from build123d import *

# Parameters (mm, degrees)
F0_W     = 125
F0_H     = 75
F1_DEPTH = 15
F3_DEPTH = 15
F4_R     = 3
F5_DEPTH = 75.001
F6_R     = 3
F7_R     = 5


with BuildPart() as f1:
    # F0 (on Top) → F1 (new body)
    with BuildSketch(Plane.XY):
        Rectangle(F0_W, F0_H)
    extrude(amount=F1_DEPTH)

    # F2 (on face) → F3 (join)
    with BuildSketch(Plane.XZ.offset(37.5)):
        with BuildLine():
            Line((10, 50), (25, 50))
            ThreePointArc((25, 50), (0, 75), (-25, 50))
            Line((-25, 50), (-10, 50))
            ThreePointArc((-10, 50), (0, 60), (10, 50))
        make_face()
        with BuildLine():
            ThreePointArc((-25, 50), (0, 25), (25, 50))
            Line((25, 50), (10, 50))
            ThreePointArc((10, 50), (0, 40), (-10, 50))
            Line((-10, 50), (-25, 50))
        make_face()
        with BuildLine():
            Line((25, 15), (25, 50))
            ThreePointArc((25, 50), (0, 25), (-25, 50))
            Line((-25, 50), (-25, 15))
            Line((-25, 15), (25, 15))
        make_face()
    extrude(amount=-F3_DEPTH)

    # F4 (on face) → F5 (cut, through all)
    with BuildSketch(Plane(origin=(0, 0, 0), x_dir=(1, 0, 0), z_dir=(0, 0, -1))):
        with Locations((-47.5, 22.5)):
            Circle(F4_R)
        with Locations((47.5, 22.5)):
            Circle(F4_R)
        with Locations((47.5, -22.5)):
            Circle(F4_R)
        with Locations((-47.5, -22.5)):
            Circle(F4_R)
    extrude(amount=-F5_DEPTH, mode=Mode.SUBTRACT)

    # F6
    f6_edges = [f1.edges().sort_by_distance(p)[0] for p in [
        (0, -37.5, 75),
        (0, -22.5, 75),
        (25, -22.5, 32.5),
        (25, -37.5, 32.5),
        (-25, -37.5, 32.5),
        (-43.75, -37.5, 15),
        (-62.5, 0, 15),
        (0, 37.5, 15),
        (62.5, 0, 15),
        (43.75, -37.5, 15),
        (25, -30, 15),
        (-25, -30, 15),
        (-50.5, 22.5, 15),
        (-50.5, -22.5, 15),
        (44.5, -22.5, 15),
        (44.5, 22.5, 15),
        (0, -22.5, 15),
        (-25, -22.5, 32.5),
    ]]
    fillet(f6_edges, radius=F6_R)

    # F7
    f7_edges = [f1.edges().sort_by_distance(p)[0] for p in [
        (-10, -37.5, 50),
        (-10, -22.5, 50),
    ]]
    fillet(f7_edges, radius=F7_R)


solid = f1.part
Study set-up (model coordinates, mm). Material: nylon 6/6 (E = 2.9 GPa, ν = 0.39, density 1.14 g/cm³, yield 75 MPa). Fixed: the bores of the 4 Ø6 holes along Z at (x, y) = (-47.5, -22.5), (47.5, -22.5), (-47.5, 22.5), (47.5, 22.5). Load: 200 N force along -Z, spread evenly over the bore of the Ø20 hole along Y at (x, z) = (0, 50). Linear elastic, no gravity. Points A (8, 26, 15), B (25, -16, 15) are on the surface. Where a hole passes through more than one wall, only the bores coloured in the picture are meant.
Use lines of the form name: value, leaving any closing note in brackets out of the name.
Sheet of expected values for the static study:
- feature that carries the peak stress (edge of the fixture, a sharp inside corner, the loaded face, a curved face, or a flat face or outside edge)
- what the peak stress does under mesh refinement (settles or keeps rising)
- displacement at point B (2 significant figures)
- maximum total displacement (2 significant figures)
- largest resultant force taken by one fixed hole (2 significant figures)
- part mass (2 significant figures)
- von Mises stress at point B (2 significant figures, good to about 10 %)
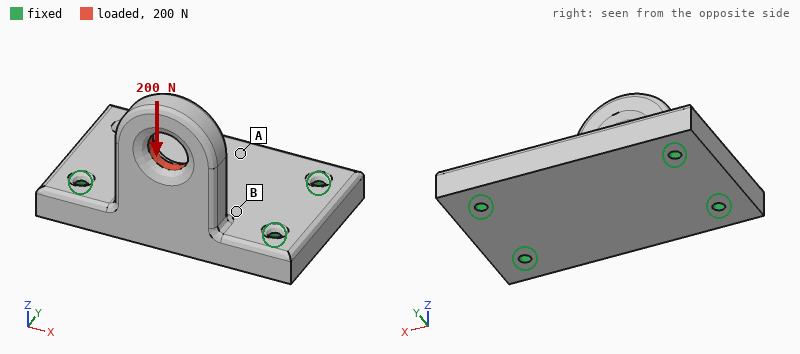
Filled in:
feature that carries the peak stress: edge of the fixture
what the peak stress does under mesh refinement: keeps rising
displacement at point B: 13 µm
maximum total displacement: 58 µm
largest resultant force taken by one fixed hole: 120 N
part mass: 200 g
von Mises stress at point B: 0.49 MPa
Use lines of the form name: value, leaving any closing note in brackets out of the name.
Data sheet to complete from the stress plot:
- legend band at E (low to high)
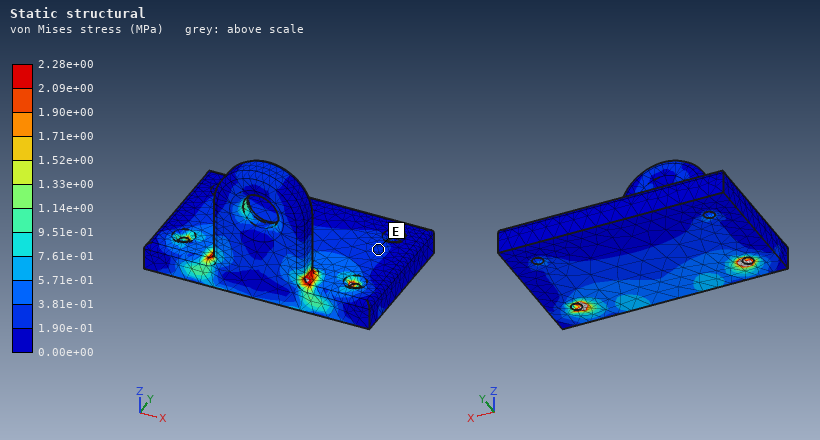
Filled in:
legend band at E: 1.90e-01 to 3.81e-01 MPa
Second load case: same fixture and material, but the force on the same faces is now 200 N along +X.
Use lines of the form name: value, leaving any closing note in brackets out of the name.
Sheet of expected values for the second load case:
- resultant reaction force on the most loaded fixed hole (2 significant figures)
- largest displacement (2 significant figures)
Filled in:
resultant reaction force on the most loaded fixed hole: 140 N
largest displacement: 76 µm
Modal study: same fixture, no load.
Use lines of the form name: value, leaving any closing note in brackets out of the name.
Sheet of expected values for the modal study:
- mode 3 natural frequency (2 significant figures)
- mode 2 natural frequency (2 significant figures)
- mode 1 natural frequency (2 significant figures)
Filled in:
mode 3 natural frequency: 1800 Hz
mode 2 natural frequency: 1700 Hz
mode 1 natural frequency: 820 Hz
